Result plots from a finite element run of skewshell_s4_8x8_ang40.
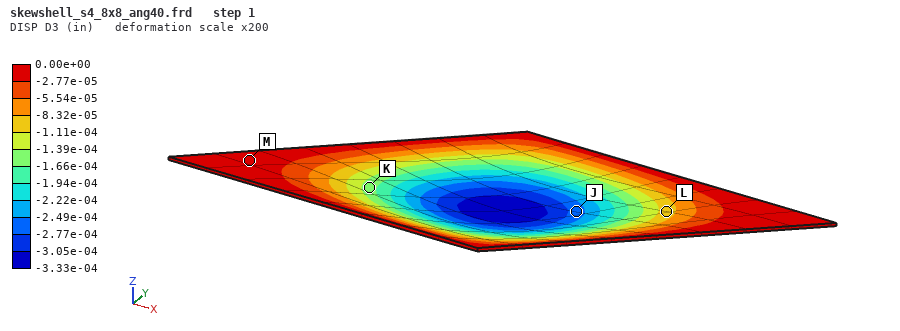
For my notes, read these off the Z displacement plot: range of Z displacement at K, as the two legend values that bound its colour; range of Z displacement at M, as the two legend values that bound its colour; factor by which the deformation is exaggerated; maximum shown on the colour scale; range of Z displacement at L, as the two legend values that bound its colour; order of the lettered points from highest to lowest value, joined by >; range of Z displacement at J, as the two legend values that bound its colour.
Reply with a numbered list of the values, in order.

1. -1.66e-04 to -1.39e-04 in
2. -2.77e-05 to 0.00e+00 in
3. 200
4. 0.00e+00 in
5. -1.11e-04 to -8.32e-05 in
6. M > L > K > J
7. -2.77e-04 to -2.49e-04 in
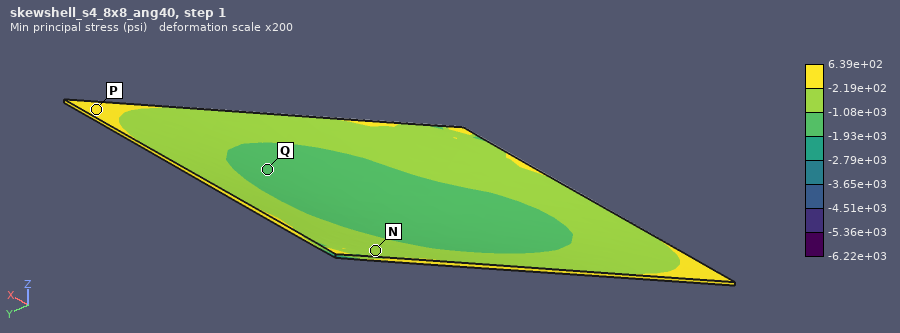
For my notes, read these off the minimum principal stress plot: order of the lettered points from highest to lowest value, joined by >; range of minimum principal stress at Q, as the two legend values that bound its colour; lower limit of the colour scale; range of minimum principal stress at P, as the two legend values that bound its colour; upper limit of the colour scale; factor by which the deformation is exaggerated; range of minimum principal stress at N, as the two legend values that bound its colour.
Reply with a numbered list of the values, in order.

1. P > N > Q
2. -1.93e+03 to -1.08e+03 psi
3. -6.22e+03 psi
4. -2.19e+02 to 6.39e+02 psi
5. 6.39e+02 psi
6. 200
7. -1.08e+03 to -2.19e+02 psi
